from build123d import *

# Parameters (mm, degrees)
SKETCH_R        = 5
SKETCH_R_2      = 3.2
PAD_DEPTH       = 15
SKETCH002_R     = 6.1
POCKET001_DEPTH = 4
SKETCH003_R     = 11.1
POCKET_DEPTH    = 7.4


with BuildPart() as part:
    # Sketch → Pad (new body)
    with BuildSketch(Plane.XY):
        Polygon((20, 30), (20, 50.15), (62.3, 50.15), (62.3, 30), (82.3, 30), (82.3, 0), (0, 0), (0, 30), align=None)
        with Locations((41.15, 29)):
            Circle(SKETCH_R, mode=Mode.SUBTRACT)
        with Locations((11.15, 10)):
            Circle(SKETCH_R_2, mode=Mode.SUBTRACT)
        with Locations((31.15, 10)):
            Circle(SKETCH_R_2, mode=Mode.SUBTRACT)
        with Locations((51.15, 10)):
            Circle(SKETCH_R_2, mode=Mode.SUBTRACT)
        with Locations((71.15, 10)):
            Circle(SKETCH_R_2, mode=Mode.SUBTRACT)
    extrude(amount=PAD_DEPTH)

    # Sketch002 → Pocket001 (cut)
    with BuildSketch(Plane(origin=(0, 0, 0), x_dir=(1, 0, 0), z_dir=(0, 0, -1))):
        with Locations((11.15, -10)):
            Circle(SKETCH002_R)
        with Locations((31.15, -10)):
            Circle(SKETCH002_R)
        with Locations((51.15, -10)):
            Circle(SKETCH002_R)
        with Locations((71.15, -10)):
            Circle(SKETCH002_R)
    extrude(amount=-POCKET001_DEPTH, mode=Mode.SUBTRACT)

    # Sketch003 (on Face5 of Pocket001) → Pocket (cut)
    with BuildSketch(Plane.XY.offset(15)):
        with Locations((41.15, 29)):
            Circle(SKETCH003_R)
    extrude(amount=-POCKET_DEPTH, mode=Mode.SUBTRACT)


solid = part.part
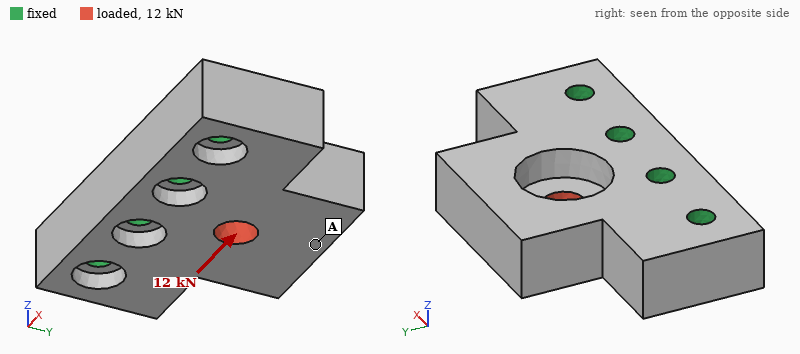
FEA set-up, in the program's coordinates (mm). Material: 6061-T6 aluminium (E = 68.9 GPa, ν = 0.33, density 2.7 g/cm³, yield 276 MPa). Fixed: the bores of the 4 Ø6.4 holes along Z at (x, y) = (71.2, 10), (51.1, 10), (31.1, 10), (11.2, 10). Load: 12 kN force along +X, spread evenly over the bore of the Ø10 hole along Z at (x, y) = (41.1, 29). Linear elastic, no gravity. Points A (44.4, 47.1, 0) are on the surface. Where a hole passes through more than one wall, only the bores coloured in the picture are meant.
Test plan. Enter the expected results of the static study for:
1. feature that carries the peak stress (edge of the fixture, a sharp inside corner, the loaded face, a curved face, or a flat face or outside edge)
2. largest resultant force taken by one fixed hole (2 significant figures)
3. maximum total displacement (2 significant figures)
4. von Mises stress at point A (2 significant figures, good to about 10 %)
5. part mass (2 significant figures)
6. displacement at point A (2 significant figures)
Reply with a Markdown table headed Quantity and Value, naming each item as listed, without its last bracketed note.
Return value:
| Quantity | Value |
|---|---|
| feature that carries the peak stress | the loaded face |
| largest resultant force taken by one fixed hole | 4.4 kN |
| maximum total displacement | 23 µm |
| von Mises stress at point A | 14 MPa |
| part mass | 120 g |
| displacement at point A | 18 µm |
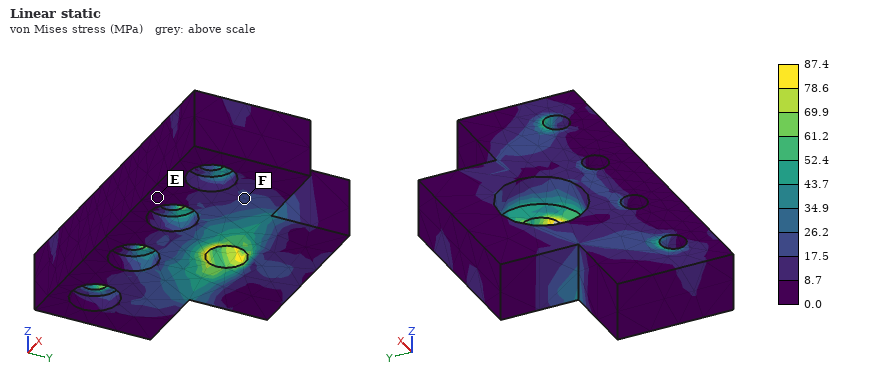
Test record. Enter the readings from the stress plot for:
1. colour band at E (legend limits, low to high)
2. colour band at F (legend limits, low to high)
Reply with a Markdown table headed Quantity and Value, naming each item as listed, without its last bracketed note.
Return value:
| Quantity | Value |
|---|---|
| colour band at E | 0.0 to 8.7 MPa |
| colour band at F | 17.5 to 26.2 MPa |
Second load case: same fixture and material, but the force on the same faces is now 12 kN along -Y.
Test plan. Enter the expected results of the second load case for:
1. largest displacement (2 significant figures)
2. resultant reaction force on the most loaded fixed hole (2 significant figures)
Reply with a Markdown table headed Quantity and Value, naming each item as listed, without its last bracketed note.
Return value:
| Quantity | Value |
|---|---|
| largest displacement | 43 µm |
| resultant reaction force on the most loaded fixed hole | 4.6 kN |
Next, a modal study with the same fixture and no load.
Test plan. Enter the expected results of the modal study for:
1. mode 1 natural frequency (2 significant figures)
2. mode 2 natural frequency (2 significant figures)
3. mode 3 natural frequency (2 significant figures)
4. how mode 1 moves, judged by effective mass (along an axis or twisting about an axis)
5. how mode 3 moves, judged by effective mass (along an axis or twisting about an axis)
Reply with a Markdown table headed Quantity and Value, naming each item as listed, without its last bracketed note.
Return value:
| Quantity | Value |
|---|---|
| mode 1 natural frequency | 6500 Hz |
| mode 2 natural frequency | 13 kHz |
| mode 3 natural frequency | 17 kHz |
| how mode 1 moves, judged by effective mass | along Z |
| how mode 3 moves, judged by effective mass | along X |
